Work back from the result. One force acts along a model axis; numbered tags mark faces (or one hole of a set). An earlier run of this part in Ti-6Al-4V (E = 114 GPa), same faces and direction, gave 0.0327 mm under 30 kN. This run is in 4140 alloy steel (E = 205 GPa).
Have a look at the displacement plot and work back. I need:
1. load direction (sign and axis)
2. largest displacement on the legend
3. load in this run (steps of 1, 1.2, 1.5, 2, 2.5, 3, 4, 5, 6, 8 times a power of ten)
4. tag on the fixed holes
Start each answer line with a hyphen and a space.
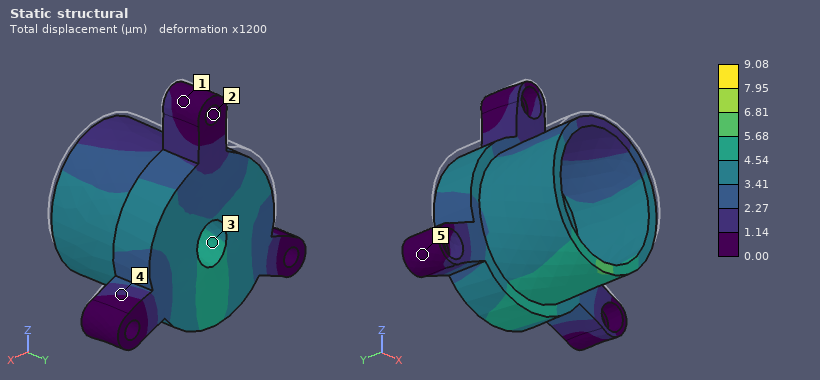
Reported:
- -Z
- 9.08 µm
- 15 kN
- 2
